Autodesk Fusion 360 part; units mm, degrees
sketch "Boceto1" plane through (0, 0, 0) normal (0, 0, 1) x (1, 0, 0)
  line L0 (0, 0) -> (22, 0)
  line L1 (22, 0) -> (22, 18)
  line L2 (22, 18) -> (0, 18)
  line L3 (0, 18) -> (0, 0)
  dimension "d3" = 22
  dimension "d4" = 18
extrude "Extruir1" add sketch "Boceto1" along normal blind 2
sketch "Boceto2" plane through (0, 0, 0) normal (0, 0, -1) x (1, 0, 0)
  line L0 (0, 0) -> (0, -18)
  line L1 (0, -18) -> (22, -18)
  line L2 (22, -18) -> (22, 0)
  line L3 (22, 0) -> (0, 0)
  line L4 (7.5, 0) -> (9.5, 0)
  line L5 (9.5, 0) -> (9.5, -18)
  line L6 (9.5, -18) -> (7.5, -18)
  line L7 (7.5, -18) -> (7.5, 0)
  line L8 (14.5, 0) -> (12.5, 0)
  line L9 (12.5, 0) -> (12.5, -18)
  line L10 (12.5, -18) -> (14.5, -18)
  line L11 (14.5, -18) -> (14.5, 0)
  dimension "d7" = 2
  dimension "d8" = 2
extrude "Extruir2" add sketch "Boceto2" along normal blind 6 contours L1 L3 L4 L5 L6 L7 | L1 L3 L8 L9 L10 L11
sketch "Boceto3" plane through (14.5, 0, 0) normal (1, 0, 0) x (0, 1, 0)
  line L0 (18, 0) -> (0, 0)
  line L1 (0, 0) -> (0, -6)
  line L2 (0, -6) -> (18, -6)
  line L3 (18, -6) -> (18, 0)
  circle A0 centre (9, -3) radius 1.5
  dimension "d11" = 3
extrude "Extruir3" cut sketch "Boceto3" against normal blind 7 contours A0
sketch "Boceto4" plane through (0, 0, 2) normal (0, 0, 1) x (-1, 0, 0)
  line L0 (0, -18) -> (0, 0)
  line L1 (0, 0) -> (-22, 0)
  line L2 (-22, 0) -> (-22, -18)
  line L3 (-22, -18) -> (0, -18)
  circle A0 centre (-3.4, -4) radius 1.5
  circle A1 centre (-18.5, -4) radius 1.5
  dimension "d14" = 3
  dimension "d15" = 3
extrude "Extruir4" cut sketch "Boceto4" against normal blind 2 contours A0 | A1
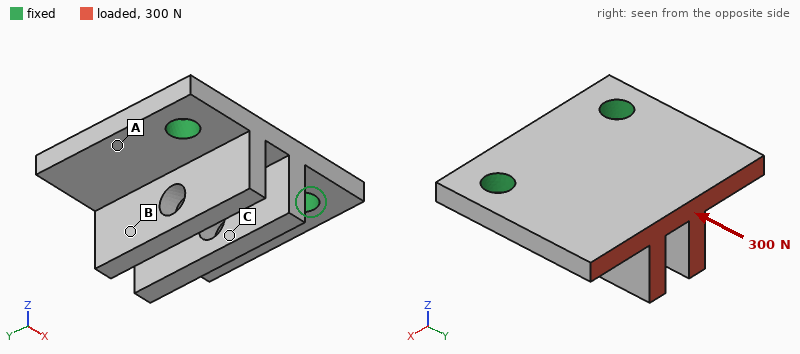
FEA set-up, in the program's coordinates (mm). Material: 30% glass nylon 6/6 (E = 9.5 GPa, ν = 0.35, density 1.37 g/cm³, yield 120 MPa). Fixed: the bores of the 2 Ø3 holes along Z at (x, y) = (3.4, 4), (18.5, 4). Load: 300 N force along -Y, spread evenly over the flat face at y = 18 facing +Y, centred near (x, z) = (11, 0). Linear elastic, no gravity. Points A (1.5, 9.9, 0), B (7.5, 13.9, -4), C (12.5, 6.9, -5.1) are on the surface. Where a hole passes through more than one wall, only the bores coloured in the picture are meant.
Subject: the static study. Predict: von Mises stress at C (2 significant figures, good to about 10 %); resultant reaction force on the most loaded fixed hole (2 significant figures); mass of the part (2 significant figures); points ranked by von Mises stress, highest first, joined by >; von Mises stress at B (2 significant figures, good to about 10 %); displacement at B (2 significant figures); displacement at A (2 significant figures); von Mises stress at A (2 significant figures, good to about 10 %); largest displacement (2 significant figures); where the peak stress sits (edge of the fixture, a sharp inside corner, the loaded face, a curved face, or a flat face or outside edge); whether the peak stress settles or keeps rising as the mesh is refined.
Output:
6.4 MPa
150 N
1.6 g
A > C > B
3.5 MPa
0.073 mm
0.020 mm
12 MPa
0.11 mm
edge of the fixture
keeps rising
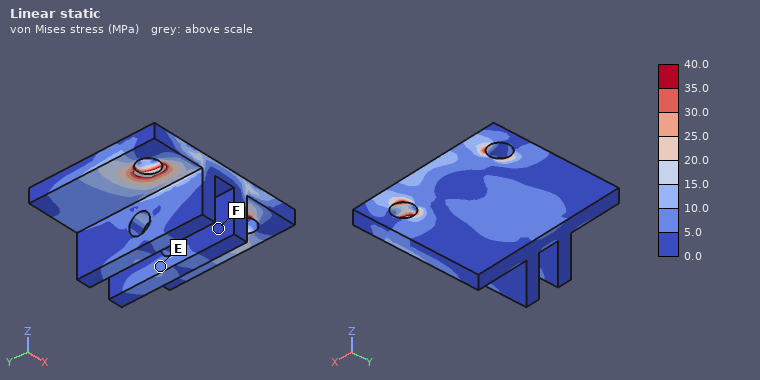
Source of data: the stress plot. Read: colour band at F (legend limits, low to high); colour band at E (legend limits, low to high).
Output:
0.0 to 5.0 MPa
5.0 to 10.0 MPa
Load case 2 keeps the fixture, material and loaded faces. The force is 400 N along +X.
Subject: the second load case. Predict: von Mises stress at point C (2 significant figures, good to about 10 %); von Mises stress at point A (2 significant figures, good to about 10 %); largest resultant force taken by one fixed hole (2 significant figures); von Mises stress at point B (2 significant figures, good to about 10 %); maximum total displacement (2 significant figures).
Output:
20 MPa
15 MPa
390 N
27 MPa
0.23 mm
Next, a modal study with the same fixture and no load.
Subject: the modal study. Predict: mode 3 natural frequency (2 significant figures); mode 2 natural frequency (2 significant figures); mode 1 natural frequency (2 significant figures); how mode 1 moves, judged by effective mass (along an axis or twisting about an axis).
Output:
12 kHz
8100 Hz
4400 Hz
along Z
